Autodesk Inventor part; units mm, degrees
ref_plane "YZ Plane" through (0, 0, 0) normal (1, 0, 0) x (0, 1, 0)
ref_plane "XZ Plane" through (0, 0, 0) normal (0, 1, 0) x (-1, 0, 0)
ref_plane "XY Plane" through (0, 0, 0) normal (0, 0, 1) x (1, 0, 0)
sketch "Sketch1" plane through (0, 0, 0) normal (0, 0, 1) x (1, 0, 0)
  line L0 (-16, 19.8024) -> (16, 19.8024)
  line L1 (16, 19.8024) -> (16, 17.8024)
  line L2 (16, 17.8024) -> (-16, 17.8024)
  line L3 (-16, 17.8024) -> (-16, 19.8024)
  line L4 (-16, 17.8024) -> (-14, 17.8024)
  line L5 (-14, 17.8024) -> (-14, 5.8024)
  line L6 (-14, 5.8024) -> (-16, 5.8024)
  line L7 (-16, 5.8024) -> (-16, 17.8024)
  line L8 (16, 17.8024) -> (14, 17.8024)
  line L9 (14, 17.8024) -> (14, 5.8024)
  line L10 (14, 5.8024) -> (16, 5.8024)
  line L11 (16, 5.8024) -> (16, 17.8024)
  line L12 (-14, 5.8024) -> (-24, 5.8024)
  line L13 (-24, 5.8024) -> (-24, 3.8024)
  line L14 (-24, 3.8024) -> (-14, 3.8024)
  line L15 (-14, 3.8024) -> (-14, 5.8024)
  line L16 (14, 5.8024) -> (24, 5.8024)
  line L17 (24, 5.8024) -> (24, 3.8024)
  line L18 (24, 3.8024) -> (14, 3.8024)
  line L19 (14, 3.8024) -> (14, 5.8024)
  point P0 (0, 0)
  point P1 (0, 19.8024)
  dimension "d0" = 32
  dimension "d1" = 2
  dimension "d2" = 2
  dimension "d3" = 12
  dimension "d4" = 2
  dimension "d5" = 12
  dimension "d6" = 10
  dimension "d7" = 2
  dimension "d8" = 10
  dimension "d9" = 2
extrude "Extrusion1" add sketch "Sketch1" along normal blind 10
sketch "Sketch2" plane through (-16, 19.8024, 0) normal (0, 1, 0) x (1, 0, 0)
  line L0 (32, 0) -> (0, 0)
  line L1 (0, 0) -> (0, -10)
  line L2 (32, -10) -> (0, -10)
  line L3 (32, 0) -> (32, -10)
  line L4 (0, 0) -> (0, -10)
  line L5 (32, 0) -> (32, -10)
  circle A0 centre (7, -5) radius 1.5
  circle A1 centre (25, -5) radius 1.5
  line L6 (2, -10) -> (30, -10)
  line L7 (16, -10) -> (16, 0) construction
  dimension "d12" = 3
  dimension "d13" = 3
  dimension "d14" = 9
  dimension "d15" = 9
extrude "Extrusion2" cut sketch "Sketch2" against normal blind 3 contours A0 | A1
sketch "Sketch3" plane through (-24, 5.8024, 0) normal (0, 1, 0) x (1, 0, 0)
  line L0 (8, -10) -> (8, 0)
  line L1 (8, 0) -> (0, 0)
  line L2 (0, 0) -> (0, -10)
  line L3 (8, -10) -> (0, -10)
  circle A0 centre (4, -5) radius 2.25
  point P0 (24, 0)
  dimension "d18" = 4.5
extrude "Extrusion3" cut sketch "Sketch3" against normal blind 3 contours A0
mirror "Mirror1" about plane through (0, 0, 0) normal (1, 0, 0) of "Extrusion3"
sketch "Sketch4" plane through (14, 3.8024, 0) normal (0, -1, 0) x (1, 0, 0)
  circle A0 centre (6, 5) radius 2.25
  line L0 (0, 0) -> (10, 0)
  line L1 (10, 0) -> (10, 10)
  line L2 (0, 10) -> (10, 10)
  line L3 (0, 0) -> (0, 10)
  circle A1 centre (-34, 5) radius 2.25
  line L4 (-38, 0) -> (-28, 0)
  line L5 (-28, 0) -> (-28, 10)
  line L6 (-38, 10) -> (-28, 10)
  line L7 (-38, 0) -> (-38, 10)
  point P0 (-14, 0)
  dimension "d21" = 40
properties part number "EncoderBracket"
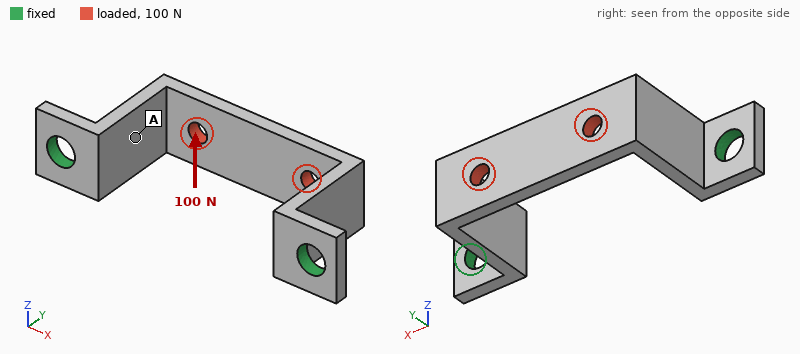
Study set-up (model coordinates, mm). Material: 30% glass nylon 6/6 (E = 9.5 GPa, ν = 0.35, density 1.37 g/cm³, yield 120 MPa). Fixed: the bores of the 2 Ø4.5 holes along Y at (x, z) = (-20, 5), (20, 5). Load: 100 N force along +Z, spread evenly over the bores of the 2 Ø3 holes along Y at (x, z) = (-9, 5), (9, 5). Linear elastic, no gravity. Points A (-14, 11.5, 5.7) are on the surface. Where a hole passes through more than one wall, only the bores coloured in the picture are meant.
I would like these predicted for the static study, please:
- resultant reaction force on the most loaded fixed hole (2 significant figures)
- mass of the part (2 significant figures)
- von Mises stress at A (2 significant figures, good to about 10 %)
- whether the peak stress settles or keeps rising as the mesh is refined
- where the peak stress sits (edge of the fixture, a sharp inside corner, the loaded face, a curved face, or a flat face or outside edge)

50 N
2.0 g
12 MPa
keeps rising
edge of the fixture
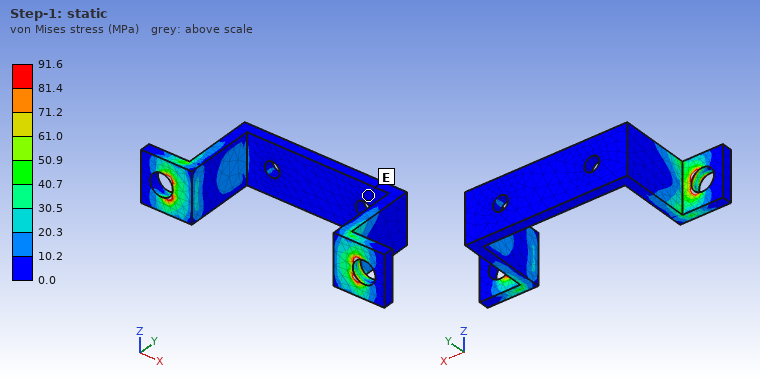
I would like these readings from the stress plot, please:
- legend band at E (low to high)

0.0 to 10.2 MPa
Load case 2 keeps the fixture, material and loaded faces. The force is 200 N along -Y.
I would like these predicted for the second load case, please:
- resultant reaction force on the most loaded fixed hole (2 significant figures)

110 N
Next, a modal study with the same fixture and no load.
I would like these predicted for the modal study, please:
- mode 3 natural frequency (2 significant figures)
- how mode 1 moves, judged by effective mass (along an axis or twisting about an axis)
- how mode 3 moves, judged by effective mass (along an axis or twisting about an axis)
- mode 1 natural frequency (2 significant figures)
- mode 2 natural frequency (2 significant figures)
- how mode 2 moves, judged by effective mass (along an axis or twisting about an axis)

4500 Hz
along X
twisting about Y
2400 Hz
3000 Hz
along Z
